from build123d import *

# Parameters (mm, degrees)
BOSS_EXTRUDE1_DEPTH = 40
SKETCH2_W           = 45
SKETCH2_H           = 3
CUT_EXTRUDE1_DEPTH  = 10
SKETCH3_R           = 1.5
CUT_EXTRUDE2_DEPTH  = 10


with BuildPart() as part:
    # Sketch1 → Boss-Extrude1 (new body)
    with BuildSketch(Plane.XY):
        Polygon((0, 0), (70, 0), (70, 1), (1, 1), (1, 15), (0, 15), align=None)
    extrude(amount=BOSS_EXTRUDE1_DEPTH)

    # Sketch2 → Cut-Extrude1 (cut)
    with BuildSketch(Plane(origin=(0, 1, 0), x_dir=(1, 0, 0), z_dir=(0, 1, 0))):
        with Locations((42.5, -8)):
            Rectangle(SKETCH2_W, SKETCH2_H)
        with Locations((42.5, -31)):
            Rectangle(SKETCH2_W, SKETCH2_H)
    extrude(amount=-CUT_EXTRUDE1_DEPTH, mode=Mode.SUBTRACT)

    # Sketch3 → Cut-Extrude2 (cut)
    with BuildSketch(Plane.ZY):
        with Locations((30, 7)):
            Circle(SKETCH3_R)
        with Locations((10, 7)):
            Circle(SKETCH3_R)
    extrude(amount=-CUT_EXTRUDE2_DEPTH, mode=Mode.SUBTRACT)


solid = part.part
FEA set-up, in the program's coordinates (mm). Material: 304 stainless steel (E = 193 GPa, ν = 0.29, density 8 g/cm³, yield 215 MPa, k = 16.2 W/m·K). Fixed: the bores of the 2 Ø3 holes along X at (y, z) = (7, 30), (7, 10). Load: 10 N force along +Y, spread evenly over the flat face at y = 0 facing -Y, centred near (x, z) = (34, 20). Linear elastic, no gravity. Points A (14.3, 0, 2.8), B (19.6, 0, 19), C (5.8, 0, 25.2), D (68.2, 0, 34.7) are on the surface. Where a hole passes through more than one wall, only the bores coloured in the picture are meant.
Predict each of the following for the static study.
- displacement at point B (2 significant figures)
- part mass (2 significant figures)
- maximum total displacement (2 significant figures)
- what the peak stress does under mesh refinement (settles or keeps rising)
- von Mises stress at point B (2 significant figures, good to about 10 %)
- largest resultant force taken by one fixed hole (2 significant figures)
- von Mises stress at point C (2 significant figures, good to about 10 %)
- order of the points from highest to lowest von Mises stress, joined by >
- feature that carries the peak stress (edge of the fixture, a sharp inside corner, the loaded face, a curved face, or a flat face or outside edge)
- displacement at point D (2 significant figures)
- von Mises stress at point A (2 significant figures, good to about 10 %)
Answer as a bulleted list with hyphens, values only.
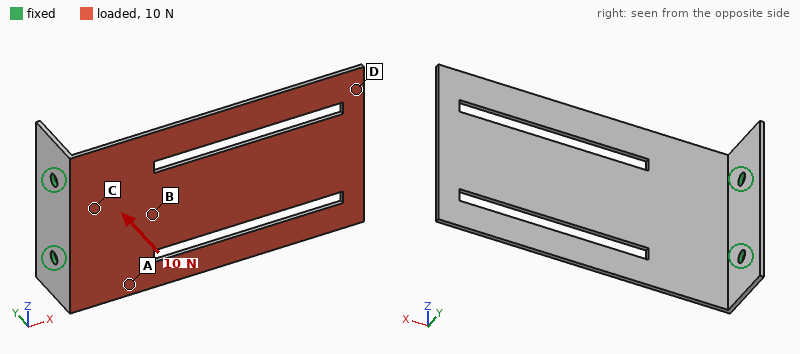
- 0.13 mm
- 25 g
- 0.84 mm
- keeps rising
- 26 MPa
- 5.1 N
- 39 MPa
- C > A > B > D
- edge of the fixture
- 0.81 mm
- 32 MPa
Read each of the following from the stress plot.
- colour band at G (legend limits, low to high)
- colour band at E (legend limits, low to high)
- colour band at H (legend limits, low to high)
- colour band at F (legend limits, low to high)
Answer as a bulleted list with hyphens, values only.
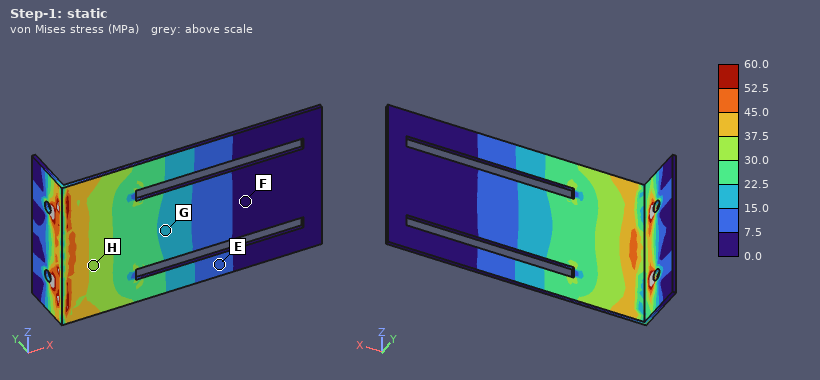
- 15.0 to 22.5 MPa
- 7.5 to 15.0 MPa
- 30.0 to 37.5 MPa
- 0.0 to 7.5 MPa
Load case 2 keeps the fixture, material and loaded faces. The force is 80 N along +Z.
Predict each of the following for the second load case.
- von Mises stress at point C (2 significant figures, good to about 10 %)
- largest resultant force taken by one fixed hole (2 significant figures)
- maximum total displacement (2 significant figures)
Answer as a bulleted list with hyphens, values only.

- 21 MPa
- 130 N
- 0.18 mm
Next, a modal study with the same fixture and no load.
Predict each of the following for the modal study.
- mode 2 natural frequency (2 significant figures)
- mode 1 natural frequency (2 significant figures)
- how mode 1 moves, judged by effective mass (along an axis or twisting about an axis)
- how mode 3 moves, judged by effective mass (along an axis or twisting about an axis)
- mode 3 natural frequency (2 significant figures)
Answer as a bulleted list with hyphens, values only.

- 580 Hz
- 150 Hz
- along Y
- along Y
- 920 Hz
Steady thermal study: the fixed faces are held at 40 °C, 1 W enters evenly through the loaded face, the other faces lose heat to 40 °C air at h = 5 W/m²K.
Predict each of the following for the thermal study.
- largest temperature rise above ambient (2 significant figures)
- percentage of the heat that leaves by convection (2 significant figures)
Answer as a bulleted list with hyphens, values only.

- 37 K
- 41 %
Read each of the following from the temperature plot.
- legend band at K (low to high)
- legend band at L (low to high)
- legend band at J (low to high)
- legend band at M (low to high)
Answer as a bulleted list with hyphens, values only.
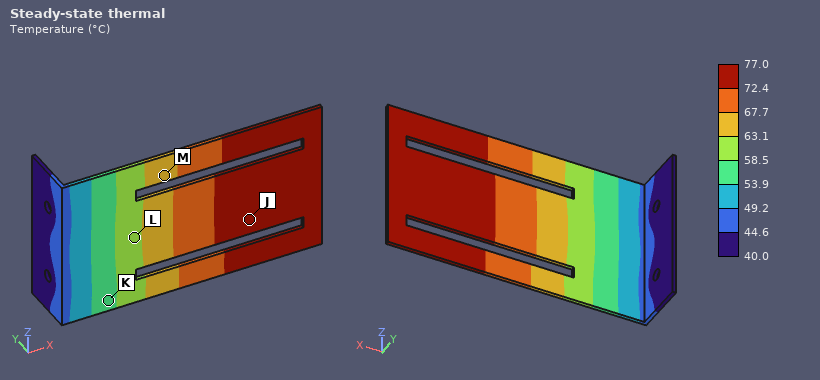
- 53.9 to 58.5 °C
- 58.5 to 63.1 °C
- 72.4 to 77.0 °C
- 63.1 to 67.7 °C
